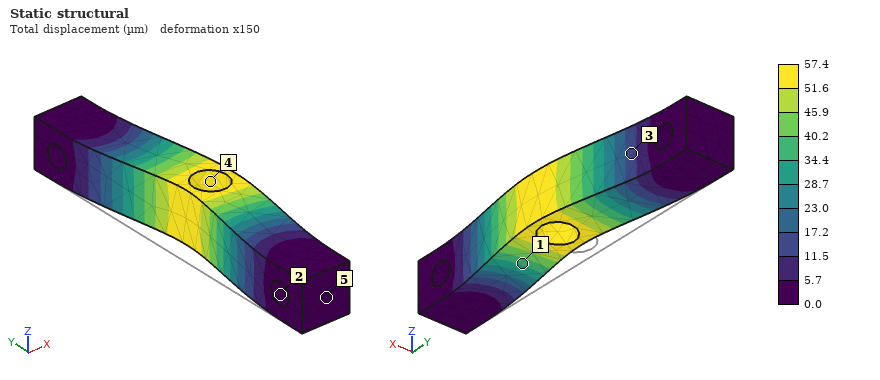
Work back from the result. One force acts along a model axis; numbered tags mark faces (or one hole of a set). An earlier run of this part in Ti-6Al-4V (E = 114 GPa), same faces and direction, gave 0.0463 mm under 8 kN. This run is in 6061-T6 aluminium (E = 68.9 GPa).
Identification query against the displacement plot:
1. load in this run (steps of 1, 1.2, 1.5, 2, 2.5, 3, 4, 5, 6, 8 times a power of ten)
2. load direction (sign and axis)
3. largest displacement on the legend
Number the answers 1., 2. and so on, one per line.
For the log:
1. 6 kN
2. +X
3. 57.4 µm
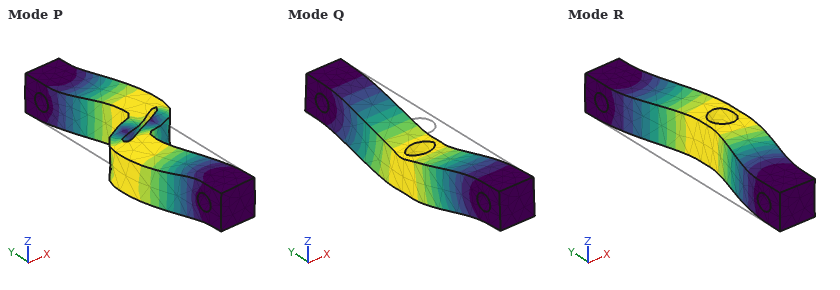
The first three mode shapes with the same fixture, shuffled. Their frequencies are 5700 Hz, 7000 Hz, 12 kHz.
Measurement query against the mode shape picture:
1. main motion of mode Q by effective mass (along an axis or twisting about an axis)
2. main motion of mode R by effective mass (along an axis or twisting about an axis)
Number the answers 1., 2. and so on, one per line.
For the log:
1. along Z
2. along X
